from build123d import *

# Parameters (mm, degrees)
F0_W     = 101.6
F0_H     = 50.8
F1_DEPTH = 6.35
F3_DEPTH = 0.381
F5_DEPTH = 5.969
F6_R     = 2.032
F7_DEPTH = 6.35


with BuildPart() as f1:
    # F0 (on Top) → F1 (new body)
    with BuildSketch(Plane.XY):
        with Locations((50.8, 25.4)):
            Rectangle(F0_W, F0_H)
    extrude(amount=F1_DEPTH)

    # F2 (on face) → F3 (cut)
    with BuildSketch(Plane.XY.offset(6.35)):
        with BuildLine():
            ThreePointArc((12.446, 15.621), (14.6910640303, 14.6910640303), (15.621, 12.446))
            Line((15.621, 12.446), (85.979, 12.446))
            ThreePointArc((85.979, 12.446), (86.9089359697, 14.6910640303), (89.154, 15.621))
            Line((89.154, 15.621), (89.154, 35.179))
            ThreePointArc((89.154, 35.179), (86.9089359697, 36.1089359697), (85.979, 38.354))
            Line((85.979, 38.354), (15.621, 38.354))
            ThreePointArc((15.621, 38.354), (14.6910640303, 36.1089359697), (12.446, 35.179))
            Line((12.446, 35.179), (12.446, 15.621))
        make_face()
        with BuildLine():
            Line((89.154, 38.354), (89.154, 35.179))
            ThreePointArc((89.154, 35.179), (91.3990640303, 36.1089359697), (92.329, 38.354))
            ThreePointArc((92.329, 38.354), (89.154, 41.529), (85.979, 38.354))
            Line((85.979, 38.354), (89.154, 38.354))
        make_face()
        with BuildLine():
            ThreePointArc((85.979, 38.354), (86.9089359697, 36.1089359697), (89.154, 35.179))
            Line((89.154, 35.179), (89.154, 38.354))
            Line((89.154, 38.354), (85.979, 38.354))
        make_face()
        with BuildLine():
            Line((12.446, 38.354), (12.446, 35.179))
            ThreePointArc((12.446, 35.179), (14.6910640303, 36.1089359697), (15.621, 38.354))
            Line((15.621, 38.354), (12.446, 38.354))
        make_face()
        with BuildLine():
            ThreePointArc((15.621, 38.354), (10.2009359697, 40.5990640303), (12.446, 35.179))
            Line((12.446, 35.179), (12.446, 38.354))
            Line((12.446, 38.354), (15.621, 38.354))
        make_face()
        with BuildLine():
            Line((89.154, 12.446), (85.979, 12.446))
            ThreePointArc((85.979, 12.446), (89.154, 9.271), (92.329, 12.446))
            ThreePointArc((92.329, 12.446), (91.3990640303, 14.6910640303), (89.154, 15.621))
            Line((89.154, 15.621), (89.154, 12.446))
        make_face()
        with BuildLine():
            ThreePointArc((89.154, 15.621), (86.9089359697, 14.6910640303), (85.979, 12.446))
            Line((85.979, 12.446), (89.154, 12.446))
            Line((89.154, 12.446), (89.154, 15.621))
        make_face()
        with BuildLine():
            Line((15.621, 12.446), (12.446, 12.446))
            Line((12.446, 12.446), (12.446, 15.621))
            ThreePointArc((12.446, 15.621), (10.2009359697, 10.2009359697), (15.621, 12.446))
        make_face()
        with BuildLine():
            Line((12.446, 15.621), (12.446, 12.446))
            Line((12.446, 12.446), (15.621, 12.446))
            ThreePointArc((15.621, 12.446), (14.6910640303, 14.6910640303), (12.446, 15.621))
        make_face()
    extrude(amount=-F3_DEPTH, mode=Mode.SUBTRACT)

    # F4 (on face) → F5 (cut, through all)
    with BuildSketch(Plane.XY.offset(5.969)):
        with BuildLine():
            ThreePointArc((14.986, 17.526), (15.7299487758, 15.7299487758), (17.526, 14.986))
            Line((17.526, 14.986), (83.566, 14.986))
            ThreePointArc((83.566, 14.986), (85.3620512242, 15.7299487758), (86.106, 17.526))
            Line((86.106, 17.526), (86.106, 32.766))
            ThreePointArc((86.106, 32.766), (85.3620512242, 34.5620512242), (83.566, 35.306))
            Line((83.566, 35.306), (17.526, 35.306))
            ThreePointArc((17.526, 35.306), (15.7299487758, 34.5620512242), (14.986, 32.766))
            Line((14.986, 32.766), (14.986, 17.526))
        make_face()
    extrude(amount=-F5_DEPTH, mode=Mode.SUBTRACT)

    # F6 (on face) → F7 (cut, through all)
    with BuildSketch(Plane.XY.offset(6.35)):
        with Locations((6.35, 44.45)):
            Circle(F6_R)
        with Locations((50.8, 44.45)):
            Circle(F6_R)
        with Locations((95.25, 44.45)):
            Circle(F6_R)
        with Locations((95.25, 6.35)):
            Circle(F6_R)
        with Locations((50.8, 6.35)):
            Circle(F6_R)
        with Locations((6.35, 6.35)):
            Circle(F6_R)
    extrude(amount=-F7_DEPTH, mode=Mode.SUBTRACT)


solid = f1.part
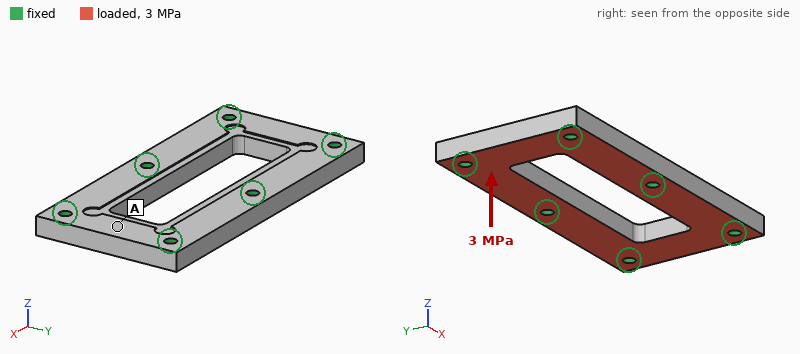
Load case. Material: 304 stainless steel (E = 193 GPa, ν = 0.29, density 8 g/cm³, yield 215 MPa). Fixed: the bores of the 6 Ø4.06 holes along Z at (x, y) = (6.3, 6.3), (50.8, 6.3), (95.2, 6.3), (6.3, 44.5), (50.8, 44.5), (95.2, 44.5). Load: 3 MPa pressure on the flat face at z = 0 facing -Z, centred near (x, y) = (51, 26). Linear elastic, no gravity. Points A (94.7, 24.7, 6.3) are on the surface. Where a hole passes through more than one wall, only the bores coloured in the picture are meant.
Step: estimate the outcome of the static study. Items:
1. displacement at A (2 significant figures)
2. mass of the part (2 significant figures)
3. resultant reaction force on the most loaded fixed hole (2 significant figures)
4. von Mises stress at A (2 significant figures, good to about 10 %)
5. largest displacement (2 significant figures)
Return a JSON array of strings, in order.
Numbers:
["5.9 µm", "180 g", "2.1 kN", "27 MPa", "11 µm"]
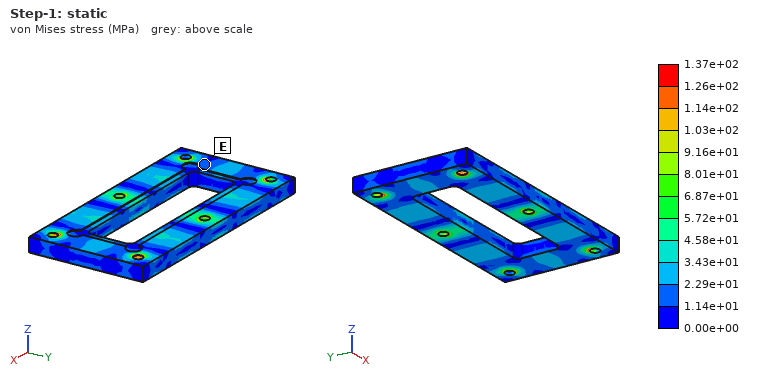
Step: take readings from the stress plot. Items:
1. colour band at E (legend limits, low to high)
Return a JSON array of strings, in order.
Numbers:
["1.14e+01 to 2.29e+01 MPa"]
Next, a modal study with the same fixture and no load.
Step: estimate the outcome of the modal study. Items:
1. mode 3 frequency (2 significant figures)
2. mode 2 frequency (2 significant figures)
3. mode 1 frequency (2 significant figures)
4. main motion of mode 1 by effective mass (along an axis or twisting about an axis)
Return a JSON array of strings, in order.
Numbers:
["15 kHz", "15 kHz", "14 kHz", "twisting about Y"]
